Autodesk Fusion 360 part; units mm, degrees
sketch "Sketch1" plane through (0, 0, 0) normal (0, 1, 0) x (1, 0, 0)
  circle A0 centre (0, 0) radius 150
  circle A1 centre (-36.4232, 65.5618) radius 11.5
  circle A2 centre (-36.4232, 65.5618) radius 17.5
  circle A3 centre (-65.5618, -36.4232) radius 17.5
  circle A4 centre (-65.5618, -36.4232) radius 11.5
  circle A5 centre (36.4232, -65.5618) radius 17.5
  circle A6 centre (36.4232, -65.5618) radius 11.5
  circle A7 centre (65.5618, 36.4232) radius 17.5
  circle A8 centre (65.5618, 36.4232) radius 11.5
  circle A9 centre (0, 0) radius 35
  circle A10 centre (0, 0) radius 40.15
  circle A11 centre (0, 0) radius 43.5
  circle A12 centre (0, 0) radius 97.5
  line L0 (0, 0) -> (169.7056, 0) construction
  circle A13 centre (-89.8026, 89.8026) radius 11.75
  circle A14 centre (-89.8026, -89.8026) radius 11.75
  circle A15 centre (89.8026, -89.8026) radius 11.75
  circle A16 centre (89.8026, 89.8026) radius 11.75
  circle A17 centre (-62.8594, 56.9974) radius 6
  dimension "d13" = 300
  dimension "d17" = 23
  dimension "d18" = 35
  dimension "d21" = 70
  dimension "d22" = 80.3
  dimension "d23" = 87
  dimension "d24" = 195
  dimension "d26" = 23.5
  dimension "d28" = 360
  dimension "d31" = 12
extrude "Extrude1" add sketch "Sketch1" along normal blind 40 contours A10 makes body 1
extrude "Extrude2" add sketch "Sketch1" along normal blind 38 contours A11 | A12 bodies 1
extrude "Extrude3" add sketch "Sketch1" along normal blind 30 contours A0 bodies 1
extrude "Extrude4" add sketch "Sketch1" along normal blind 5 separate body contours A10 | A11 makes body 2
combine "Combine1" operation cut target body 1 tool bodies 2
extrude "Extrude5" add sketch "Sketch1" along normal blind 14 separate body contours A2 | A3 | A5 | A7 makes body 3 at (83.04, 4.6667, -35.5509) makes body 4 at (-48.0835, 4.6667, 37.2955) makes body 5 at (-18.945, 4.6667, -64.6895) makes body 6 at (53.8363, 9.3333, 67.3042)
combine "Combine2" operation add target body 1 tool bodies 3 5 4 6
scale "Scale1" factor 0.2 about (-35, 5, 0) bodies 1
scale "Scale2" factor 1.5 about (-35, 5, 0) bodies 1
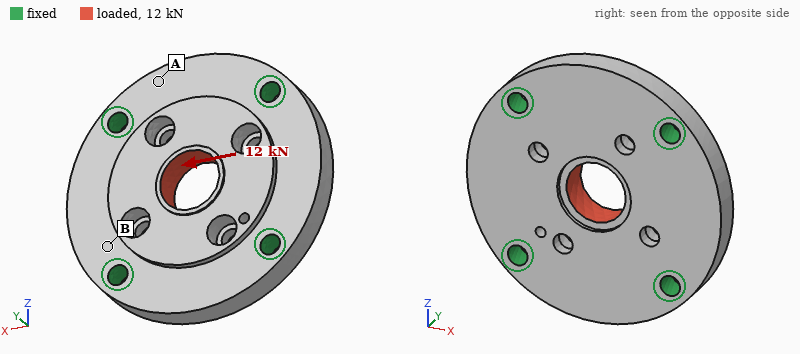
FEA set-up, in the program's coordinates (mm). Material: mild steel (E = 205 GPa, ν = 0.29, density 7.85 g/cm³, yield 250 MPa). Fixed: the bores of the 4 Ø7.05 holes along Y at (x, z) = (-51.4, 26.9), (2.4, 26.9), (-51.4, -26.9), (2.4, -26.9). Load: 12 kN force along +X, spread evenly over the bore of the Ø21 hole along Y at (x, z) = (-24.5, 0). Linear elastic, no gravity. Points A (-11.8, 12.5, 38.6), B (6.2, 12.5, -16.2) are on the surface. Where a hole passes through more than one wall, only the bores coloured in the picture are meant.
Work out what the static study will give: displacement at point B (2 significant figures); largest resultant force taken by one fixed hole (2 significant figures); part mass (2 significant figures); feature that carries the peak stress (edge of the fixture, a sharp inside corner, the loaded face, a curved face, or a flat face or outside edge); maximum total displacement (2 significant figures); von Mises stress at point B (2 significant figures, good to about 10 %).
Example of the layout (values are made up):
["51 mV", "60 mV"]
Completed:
["1.3 µm", "3.3 kN", "430 g", "a curved face", "4.6 µm", "11 MPa"]
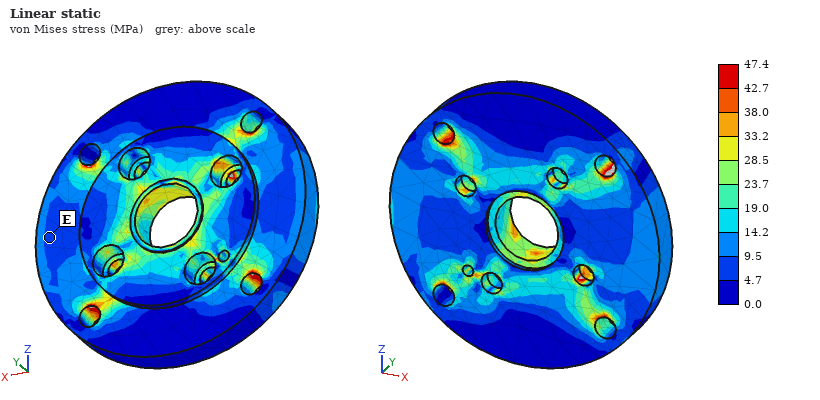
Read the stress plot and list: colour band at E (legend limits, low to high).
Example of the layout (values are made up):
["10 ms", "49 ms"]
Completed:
["4.7 to 9.5 MPa"]
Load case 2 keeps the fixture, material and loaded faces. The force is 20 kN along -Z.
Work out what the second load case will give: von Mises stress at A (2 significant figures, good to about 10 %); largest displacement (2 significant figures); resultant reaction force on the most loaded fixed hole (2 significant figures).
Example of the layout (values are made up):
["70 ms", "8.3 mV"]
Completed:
["15 MPa", "7.6 µm", "5.5 kN"]
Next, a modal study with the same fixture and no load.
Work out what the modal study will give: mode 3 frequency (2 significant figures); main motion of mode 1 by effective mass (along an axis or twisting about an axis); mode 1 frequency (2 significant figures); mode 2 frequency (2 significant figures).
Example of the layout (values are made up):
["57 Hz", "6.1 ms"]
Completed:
["13 kHz", "along Y", "12 kHz", "12 kHz"]
